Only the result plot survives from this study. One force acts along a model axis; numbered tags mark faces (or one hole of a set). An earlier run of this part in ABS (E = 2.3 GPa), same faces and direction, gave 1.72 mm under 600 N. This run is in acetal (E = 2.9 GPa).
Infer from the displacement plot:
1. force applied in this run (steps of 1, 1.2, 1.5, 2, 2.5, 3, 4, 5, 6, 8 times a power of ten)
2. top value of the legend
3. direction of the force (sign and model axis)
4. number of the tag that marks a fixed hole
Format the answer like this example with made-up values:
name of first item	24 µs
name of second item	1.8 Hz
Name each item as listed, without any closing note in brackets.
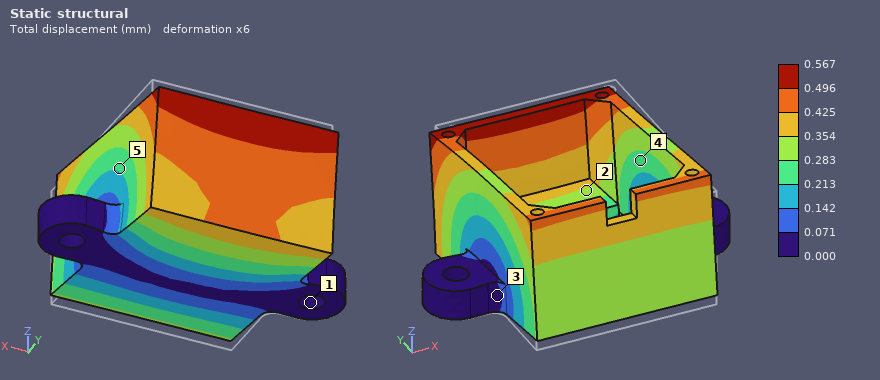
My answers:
force applied in this run	250 N
top value of the legend	0.567 mm
direction of the force	-Z
number of the tag that marks a fixed hole	1
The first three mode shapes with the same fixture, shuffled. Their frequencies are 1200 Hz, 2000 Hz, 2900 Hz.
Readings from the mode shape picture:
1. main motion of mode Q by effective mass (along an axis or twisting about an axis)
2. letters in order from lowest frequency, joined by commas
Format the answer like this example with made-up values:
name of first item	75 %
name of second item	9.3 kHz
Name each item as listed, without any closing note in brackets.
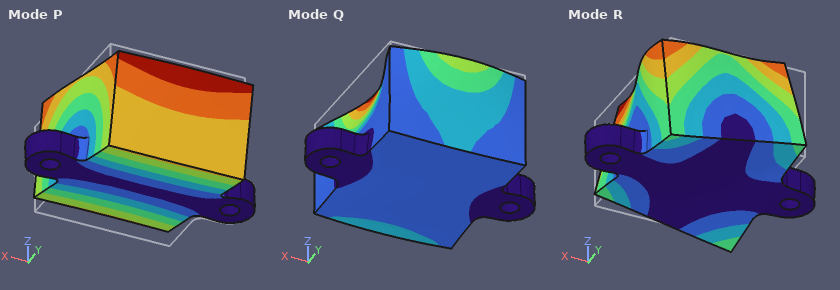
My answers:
main motion of mode Q by effective mass	along Z
letters in order from lowest frequency, joined by commas	P, R, Q
